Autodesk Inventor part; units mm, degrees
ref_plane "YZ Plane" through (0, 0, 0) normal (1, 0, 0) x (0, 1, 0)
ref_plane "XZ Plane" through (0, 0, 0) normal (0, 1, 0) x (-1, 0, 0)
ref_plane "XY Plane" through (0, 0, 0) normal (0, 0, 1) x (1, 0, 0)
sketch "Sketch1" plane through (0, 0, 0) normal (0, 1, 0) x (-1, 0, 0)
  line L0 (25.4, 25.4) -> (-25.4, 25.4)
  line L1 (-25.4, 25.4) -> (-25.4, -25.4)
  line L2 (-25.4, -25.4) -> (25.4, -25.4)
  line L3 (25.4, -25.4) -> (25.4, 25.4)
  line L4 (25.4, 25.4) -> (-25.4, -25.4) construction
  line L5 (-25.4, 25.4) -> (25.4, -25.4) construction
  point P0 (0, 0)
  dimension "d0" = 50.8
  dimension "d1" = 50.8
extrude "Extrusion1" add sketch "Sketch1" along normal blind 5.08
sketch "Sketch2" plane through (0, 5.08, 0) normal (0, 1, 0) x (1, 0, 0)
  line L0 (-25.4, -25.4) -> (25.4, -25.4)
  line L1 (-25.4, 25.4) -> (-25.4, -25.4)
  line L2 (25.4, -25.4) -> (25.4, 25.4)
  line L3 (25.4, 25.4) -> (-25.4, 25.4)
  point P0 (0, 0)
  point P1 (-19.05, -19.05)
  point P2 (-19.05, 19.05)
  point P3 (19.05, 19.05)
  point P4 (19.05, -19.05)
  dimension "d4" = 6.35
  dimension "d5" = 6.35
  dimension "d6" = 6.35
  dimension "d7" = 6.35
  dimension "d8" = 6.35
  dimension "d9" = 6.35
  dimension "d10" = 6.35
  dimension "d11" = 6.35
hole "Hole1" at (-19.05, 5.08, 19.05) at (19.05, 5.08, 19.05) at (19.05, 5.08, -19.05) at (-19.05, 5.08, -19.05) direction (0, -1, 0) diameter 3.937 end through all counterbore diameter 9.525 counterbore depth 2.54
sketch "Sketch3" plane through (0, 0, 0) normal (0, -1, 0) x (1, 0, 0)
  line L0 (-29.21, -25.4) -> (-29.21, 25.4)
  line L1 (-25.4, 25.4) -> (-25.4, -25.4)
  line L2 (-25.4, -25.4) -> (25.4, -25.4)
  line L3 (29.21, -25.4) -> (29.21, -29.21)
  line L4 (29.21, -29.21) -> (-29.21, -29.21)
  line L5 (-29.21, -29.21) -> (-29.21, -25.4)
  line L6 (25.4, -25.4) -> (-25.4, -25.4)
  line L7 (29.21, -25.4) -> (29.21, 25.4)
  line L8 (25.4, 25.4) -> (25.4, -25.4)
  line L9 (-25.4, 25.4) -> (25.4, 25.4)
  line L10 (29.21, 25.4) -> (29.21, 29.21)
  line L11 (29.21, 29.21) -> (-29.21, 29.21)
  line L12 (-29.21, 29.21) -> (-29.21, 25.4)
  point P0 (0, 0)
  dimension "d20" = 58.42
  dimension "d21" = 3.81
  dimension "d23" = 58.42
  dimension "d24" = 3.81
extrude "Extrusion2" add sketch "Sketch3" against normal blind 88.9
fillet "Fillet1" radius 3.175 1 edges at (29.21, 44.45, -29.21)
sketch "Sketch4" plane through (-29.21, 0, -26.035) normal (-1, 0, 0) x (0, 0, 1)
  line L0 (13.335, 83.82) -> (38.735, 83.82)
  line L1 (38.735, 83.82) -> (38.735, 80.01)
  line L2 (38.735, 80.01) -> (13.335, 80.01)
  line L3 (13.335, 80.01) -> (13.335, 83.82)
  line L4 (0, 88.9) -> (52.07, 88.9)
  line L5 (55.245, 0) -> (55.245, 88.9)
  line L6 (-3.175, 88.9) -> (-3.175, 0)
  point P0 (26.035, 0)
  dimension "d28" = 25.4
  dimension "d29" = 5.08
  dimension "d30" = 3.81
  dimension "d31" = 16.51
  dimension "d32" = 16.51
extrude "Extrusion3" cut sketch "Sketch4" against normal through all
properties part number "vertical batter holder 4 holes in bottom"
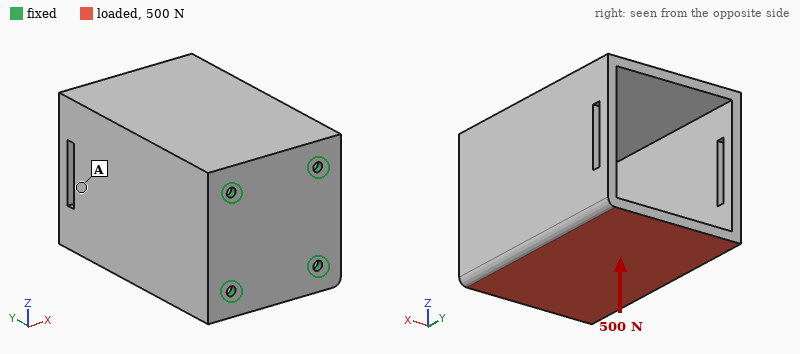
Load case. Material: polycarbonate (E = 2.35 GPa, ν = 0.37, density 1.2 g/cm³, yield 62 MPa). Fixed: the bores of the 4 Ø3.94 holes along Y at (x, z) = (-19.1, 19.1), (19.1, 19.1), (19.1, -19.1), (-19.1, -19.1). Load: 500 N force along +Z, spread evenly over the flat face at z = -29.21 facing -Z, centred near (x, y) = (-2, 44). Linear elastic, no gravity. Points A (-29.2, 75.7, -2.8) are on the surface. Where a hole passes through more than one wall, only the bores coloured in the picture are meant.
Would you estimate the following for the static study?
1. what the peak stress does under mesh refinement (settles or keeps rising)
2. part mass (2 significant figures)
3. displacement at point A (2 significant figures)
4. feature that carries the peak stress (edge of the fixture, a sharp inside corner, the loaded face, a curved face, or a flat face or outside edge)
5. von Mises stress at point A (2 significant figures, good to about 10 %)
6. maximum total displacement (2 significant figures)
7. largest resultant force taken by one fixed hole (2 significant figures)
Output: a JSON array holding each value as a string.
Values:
["keeps rising", "100 g", "0.49 mm", "edge of the fixture", "2.5 MPa", "1.1 mm", "310 N"]
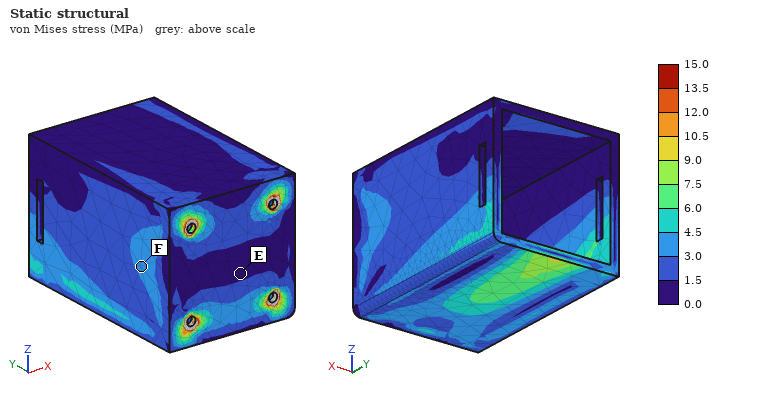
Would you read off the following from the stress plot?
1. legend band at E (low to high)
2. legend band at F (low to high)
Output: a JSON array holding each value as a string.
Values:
["0.0 to 1.5 MPa", "3.0 to 4.5 MPa"]
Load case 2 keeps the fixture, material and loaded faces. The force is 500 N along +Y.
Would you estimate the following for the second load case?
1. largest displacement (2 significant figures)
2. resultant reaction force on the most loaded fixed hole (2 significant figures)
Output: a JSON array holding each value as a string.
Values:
["0.37 mm", "320 N"]
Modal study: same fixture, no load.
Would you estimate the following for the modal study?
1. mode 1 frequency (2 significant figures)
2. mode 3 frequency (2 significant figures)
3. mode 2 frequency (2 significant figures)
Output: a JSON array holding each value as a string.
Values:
["610 Hz", "690 Hz", "610 Hz"]
